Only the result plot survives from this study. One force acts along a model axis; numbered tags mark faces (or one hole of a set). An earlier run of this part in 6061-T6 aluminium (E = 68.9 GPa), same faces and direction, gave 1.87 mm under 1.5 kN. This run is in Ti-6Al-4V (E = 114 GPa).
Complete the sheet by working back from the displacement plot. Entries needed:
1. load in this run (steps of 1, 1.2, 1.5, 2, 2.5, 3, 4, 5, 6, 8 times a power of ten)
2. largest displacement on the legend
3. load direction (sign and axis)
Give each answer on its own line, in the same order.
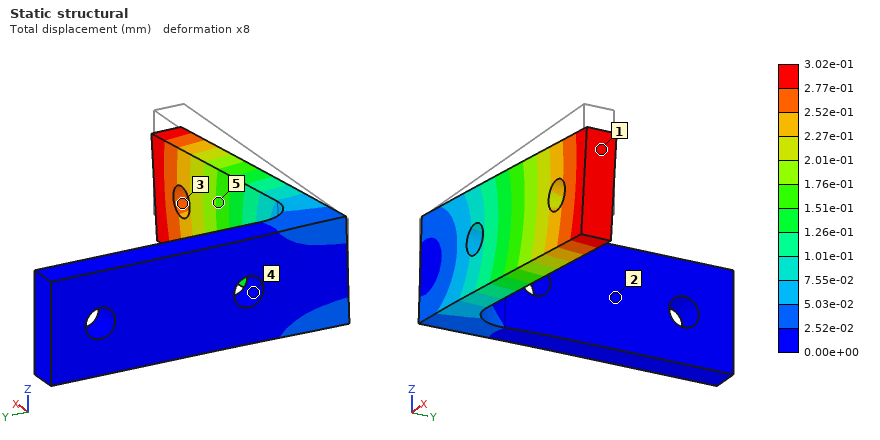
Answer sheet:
400 N
3.02e-01 mm
-Z
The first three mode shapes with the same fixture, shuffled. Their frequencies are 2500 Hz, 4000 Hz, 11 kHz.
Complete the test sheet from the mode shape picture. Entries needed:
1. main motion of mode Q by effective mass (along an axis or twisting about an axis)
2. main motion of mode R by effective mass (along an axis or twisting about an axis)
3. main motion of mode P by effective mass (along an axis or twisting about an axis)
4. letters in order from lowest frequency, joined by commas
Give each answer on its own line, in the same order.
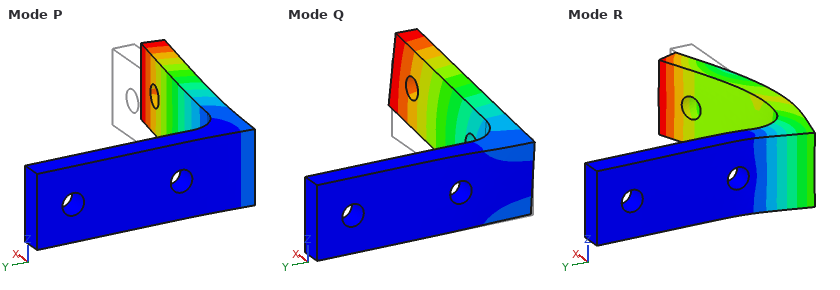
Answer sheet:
along Z
along X
along Y
P, Q, R
